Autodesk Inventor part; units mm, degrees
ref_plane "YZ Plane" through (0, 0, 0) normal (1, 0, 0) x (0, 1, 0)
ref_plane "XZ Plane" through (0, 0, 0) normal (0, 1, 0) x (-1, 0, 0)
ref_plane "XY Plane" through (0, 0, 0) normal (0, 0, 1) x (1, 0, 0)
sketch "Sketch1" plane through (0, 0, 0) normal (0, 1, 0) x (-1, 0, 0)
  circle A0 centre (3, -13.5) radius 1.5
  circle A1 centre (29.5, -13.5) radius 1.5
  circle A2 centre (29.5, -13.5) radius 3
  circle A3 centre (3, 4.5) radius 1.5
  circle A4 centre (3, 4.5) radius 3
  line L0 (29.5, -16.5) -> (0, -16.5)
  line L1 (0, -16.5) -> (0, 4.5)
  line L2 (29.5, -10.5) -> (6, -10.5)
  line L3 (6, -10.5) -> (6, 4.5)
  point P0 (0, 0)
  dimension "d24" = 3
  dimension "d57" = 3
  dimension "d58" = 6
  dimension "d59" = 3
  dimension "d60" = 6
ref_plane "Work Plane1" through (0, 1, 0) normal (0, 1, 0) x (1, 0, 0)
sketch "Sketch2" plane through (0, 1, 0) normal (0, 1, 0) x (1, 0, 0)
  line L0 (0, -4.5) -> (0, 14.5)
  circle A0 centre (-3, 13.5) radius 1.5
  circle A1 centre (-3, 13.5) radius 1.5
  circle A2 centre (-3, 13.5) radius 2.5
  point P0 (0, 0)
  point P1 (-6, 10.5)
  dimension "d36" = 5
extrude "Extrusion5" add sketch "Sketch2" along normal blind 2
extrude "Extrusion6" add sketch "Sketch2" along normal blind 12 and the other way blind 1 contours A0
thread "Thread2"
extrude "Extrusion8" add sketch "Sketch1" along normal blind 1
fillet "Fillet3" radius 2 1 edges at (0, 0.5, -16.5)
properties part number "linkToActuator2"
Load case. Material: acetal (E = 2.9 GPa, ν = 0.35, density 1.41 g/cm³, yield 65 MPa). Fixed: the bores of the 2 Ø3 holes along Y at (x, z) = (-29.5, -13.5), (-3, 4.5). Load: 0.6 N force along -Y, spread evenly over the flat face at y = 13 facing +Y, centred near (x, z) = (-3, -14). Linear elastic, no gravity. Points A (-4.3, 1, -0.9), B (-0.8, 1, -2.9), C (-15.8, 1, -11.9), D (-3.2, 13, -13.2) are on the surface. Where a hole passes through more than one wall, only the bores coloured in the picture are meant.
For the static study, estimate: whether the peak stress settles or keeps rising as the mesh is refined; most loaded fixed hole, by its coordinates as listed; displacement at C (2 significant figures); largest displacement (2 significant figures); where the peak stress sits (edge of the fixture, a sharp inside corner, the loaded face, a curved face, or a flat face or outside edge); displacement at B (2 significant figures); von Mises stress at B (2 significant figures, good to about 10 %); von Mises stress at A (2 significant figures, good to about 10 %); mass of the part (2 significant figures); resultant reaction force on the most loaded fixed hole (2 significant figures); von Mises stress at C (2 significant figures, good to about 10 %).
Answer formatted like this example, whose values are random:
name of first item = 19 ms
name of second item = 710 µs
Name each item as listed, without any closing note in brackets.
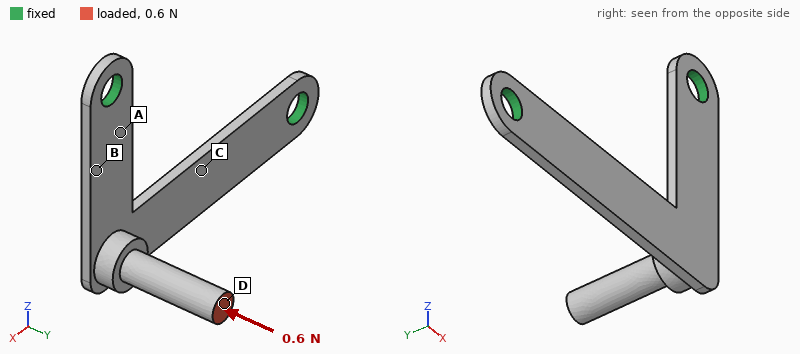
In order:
whether the peak stress settles or keeps rising as the mesh is refined = keeps rising
most loaded fixed hole, by its coordinates as listed = (-3, 4.5)
displacement at C = 0.088 mm
largest displacement = 0.44 mm
where the peak stress sits = edge of the fixture
displacement at B = 0.067 mm
von Mises stress at B = 3.1 MPa
von Mises stress at A = 3.7 MPa
mass of the part = 0.55 g
resultant reaction force on the most loaded fixed hole = 0.43 N
von Mises stress at C = 1.8 MPa
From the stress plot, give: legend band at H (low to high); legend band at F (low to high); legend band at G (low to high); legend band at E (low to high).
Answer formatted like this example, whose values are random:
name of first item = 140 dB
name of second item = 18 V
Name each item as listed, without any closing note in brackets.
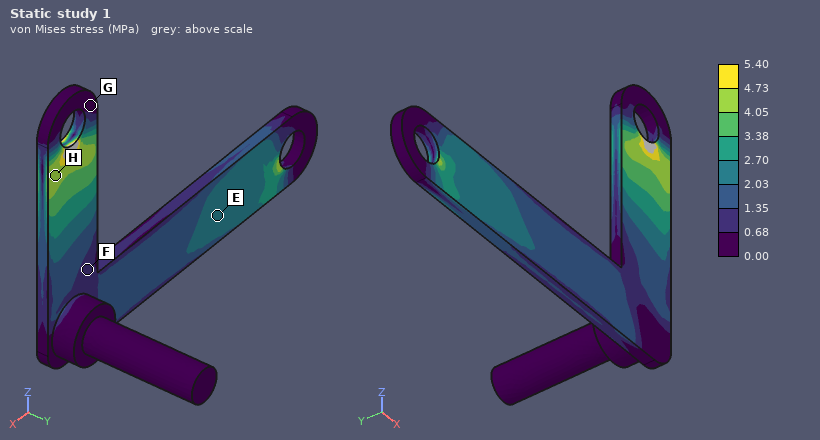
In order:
legend band at H = 4.05 to 4.73 MPa
legend band at F = 0.68 to 1.35 MPa
legend band at G = 0.00 to 0.68 MPa
legend band at E = 2.03 to 2.70 MPa
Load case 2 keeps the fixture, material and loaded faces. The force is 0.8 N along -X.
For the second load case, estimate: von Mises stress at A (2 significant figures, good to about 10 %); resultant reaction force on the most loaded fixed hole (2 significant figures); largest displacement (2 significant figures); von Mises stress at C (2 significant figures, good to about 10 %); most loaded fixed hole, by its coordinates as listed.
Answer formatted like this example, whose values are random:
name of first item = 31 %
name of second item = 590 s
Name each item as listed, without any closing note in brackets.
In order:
von Mises stress at A = 4.5 MPa
resultant reaction force on the most loaded fixed hole = 0.85 N
largest displacement = 0.51 mm
von Mises stress at C = 2.6 MPa
most loaded fixed hole, by its coordinates as listed = (-29.5, -13.5)
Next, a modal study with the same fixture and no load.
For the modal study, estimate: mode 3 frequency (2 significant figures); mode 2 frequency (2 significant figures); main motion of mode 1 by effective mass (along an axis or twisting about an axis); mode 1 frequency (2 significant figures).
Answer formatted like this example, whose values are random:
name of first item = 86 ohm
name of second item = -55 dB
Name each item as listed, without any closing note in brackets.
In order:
mode 3 frequency = 1500 Hz
mode 2 frequency = 1100 Hz
main motion of mode 1 by effective mass = along Y
mode 1 frequency = 410 Hz
